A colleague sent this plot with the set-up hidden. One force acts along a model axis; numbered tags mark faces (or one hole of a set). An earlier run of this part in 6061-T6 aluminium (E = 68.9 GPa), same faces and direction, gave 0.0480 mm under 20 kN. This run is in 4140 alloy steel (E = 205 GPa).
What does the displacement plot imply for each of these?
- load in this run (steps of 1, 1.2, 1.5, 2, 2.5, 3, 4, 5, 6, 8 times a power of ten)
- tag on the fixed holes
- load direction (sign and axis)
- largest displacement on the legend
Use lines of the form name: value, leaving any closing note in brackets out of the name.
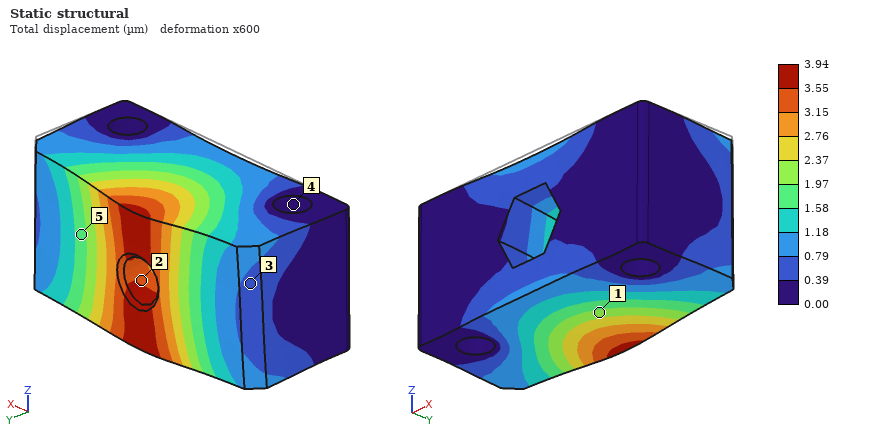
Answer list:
load in this run: 5 kN
tag on the fixed holes: 4
load direction: -Z
largest displacement on the legend: 3.94 µm
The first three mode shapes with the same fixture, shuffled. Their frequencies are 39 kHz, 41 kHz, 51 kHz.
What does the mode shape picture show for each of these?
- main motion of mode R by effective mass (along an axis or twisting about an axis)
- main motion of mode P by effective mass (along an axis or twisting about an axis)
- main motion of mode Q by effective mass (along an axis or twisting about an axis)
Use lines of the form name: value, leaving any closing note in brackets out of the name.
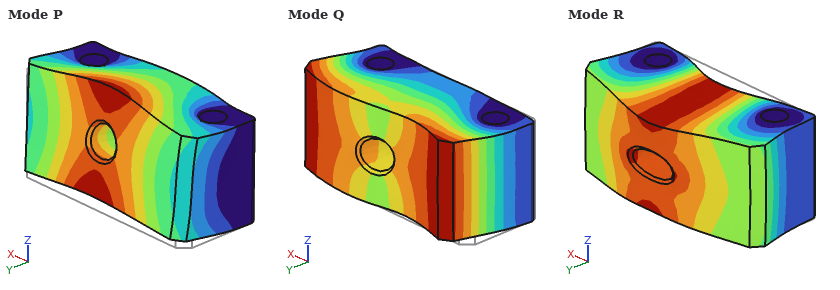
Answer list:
main motion of mode R by effective mass: along Y
main motion of mode P by effective mass: along Z
main motion of mode Q by effective mass: along X
